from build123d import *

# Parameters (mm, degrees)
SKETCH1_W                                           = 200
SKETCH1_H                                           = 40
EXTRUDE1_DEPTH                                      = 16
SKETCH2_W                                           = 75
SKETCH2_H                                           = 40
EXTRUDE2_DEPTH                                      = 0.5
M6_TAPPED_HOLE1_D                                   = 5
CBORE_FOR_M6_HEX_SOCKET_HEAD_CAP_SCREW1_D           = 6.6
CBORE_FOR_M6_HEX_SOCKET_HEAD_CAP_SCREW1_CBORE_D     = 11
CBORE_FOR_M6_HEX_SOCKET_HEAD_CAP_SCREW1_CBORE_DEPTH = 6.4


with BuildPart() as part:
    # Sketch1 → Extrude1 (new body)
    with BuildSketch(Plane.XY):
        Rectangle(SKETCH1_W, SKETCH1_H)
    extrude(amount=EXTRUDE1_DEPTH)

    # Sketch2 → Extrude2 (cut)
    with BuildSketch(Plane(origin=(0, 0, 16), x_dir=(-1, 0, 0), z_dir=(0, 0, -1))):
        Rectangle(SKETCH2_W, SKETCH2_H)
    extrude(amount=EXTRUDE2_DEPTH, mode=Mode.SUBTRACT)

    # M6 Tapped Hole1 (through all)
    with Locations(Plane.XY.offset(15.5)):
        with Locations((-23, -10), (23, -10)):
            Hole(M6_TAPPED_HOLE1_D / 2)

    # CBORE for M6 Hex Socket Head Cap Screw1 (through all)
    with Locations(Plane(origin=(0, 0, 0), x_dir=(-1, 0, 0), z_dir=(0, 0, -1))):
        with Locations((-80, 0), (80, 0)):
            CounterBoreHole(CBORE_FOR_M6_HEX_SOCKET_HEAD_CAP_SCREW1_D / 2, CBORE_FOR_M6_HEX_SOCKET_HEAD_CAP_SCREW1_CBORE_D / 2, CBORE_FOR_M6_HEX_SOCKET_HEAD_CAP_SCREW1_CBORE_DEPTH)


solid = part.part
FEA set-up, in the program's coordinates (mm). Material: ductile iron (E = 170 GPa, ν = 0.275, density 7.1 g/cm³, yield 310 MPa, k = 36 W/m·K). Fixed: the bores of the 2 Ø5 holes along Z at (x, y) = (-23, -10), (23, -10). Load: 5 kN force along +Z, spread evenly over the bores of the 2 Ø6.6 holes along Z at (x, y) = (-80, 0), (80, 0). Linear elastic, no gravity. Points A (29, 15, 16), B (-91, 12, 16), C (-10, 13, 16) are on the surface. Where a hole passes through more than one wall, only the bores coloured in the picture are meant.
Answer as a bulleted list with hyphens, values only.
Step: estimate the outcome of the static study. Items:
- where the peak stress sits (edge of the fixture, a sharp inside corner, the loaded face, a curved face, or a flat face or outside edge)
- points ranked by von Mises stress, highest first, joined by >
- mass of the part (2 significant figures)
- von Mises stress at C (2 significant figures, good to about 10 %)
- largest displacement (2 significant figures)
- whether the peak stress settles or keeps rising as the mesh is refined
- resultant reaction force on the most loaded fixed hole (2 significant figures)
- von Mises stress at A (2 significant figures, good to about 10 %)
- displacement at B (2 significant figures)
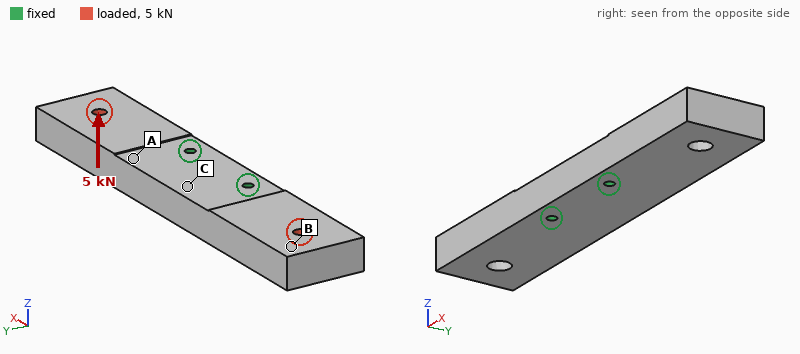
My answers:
- edge of the fixture
- A > C > B
- 880 g
- 37 MPa
- 0.15 mm
- keeps rising
- 2.5 kN
- 56 MPa
- 0.13 mm
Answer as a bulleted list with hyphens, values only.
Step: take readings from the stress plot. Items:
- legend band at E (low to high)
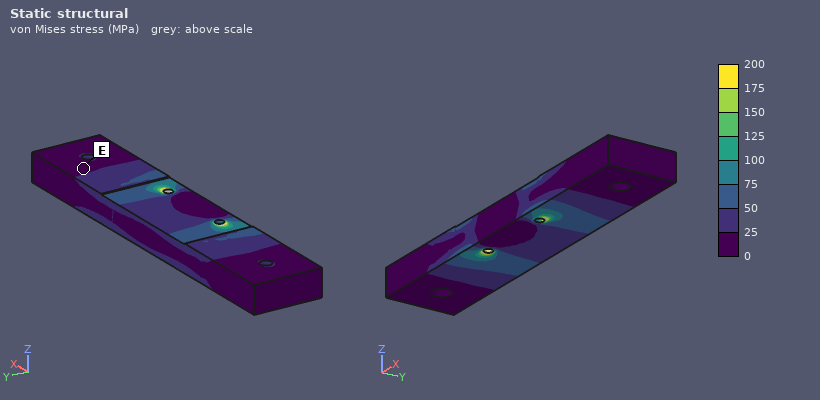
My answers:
- 0 to 25 MPa
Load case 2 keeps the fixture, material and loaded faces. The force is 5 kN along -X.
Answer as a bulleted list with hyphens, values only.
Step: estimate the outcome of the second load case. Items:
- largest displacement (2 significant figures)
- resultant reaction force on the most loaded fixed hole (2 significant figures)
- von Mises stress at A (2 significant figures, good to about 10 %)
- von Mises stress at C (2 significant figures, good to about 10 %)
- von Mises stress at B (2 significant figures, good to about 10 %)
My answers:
- 13 µm
- 2.7 kN
- 8.1 MPa
- 4.0 MPa
- 2.7 MPa
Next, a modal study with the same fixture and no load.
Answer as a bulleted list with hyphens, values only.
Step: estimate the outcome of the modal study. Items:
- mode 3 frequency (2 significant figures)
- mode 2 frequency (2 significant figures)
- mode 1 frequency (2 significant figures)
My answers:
- 3100 Hz
- 1800 Hz
- 1800 Hz
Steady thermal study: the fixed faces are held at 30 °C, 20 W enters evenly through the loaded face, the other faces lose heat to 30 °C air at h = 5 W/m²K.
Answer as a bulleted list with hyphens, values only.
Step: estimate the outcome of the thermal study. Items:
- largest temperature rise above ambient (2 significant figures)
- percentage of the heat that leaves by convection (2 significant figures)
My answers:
- 32 K
- 9.2 %
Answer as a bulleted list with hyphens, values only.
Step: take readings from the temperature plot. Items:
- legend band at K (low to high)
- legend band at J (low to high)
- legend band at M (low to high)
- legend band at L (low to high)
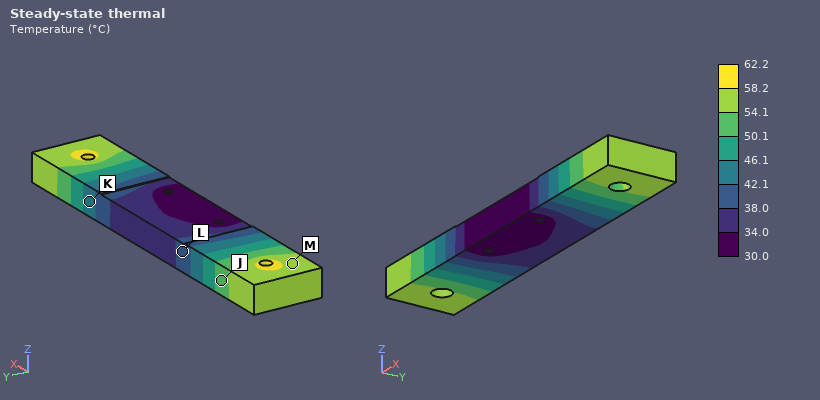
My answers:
- 42.1 to 46.1 °C
- 50.1 to 54.1 °C
- 54.1 to 58.2 °C
- 38.0 to 42.1 °C
